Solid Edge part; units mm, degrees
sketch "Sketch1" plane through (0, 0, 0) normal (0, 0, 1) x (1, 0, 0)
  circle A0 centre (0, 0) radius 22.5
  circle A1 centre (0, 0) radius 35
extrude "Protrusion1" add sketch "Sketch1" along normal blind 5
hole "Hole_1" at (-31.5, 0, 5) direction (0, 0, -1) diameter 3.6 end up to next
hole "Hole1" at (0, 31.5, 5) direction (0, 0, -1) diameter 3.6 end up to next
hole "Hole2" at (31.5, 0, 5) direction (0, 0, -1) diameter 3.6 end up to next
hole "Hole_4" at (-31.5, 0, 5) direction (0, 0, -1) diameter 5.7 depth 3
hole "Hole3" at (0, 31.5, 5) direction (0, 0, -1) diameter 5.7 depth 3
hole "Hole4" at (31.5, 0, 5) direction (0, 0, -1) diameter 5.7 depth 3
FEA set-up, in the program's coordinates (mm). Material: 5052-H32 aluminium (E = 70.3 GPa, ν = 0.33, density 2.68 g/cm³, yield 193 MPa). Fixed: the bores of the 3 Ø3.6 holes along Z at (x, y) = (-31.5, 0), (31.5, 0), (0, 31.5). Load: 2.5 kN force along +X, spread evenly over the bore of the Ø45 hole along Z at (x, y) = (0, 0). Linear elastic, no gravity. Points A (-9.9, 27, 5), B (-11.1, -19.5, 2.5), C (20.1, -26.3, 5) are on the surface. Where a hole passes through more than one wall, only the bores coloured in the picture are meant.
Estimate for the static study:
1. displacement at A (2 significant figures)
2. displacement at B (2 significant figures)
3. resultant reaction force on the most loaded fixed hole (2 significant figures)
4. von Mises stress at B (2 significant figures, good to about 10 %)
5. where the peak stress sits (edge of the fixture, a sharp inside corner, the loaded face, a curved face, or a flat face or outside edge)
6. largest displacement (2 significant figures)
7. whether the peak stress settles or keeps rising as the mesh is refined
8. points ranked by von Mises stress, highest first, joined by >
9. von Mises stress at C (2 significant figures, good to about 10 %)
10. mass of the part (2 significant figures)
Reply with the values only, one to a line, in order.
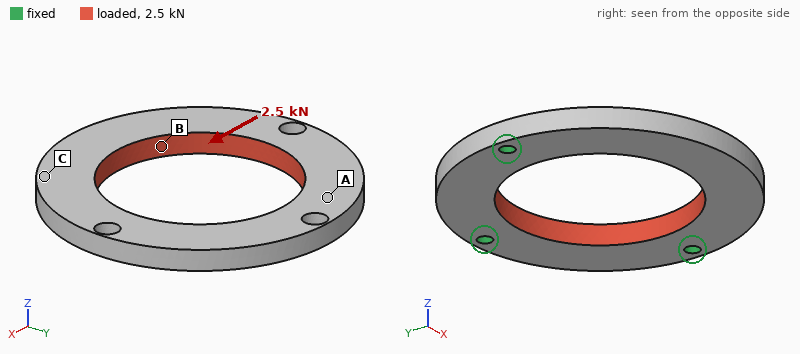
5.4 µm
22 µm
970 N
30 MPa
edge of the fixture
24 µm
keeps rising
B > C > A
15 MPa
29 g
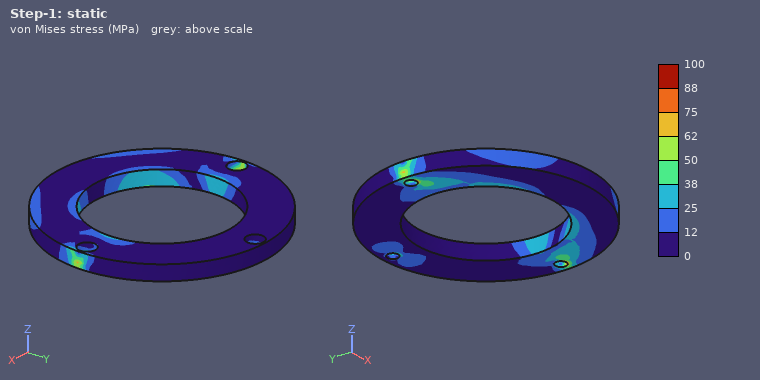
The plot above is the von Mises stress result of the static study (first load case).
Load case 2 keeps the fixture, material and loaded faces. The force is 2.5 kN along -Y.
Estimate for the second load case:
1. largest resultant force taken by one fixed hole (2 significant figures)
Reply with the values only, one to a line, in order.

1.0 kN
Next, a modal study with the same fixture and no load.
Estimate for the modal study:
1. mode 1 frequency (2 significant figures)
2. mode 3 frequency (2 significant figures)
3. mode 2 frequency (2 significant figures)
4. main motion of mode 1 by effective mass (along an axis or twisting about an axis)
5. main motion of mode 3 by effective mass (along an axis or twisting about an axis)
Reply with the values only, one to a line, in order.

1900 Hz
7700 Hz
5500 Hz
along Z
twisting about Y
